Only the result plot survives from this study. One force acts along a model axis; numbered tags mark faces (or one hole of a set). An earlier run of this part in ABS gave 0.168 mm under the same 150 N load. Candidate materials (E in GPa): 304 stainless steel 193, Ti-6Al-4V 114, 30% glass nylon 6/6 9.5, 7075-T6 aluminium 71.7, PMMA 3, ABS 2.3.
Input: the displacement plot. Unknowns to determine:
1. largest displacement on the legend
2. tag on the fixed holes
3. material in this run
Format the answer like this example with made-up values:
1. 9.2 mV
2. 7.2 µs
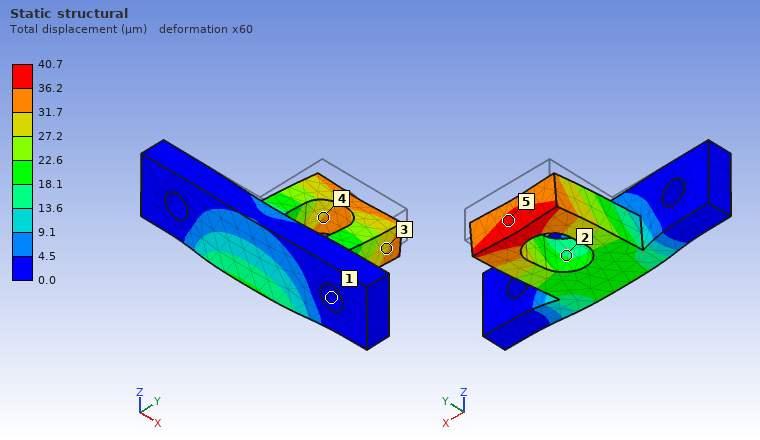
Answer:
1. 40.7 µm
2. 1
3. 30% glass nylon 6/6
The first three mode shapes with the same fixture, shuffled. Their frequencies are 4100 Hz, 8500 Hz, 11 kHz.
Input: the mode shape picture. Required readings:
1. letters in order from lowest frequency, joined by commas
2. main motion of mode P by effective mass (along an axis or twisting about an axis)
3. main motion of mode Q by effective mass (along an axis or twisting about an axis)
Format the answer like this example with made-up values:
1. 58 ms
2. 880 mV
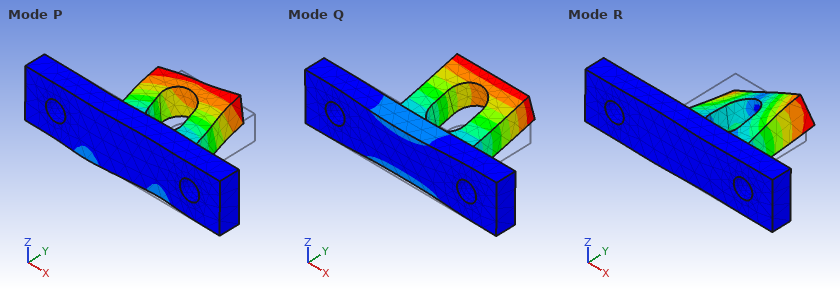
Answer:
1. Q, P, R
2. along X
3. along Z
